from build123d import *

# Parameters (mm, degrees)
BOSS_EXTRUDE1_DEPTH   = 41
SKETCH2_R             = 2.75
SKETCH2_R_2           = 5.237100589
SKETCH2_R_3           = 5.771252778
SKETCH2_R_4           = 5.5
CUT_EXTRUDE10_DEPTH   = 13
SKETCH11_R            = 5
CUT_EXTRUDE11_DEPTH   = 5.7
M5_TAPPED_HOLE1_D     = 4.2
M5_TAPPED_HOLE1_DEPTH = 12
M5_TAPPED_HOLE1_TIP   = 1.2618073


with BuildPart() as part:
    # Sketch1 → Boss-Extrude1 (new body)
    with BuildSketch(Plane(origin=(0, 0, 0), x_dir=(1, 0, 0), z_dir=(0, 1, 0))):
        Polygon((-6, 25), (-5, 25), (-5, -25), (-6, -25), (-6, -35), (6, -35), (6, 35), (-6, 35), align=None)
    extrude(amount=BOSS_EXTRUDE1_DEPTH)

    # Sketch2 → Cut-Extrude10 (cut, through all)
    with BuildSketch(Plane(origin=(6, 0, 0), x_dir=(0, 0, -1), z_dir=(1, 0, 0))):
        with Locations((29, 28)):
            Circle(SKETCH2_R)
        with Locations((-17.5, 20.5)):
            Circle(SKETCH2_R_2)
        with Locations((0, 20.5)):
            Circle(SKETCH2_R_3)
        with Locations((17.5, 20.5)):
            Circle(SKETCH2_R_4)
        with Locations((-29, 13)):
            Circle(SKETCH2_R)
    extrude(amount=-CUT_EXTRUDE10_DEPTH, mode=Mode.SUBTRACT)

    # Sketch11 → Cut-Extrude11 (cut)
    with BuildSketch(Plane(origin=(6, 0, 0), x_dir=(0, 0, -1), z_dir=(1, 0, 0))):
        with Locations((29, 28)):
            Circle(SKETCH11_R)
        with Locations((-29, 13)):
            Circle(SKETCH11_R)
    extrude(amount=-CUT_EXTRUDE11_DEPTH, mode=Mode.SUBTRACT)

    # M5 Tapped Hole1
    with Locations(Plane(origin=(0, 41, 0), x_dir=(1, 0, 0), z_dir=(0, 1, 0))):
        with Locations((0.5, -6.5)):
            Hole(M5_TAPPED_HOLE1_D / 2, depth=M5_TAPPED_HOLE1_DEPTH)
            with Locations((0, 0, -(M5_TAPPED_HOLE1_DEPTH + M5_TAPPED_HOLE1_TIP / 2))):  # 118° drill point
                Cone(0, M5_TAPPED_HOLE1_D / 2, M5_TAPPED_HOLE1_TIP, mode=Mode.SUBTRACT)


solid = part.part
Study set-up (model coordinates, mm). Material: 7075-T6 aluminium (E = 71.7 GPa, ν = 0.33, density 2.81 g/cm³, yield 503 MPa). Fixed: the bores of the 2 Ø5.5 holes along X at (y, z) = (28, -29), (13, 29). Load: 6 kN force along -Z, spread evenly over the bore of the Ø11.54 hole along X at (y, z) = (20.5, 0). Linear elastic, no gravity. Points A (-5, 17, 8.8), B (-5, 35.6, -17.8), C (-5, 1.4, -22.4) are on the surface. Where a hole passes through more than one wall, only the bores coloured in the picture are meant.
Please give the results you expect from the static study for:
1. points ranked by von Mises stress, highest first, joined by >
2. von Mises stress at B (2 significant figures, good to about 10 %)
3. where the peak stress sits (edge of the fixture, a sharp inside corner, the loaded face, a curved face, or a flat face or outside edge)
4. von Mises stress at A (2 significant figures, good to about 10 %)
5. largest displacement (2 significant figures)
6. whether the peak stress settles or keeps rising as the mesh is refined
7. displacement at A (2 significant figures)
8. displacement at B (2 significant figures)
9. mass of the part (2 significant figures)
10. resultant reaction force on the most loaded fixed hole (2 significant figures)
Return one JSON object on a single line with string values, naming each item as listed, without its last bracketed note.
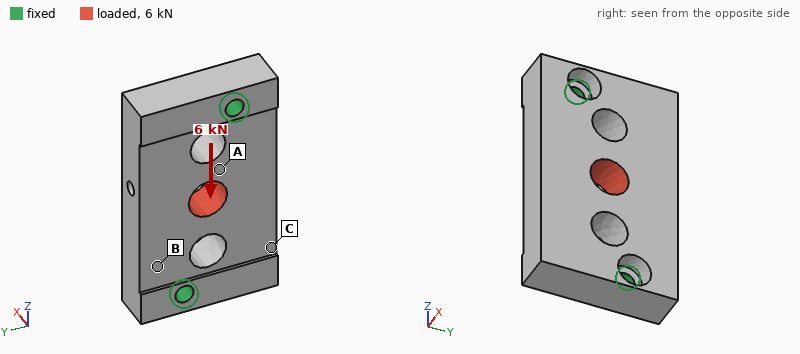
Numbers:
{"points ranked by von Mises stress, highest first, joined by >": "A > B > C", "von Mises stress at B": "16 MPa", "where the peak stress sits": "edge of the fixture", "von Mises stress at A": "25 MPa", "largest displacement": "13 µm", "whether the peak stress settles or keeps rising as the mesh is refined": "keeps rising", "displacement at A": "9.8 µm", "displacement at B": "6.1 µm", "mass of the part": "78 g", "resultant reaction force on the most loaded fixed hole": "3.0 kN"}
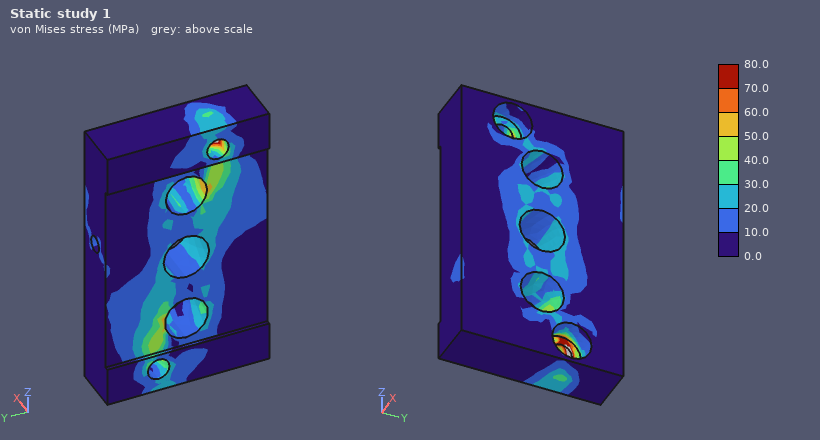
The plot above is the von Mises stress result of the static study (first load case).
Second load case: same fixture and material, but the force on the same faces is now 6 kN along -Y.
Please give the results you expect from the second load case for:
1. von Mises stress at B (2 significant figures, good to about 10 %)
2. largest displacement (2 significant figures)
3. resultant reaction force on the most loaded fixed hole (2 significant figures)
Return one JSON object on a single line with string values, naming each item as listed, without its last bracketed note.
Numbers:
{"von Mises stress at B": "18 MPa", "largest displacement": "34 µm", "resultant reaction force on the most loaded fixed hole": "3.0 kN"}
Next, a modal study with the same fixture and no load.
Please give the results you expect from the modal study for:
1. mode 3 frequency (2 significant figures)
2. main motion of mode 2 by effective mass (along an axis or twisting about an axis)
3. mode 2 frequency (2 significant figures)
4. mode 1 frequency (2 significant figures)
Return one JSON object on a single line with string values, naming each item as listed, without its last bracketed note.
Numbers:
{"mode 3 frequency": "12 kHz", "main motion of mode 2 by effective mass": "along X", "mode 2 frequency": "7500 Hz", "mode 1 frequency": "5400 Hz"}
